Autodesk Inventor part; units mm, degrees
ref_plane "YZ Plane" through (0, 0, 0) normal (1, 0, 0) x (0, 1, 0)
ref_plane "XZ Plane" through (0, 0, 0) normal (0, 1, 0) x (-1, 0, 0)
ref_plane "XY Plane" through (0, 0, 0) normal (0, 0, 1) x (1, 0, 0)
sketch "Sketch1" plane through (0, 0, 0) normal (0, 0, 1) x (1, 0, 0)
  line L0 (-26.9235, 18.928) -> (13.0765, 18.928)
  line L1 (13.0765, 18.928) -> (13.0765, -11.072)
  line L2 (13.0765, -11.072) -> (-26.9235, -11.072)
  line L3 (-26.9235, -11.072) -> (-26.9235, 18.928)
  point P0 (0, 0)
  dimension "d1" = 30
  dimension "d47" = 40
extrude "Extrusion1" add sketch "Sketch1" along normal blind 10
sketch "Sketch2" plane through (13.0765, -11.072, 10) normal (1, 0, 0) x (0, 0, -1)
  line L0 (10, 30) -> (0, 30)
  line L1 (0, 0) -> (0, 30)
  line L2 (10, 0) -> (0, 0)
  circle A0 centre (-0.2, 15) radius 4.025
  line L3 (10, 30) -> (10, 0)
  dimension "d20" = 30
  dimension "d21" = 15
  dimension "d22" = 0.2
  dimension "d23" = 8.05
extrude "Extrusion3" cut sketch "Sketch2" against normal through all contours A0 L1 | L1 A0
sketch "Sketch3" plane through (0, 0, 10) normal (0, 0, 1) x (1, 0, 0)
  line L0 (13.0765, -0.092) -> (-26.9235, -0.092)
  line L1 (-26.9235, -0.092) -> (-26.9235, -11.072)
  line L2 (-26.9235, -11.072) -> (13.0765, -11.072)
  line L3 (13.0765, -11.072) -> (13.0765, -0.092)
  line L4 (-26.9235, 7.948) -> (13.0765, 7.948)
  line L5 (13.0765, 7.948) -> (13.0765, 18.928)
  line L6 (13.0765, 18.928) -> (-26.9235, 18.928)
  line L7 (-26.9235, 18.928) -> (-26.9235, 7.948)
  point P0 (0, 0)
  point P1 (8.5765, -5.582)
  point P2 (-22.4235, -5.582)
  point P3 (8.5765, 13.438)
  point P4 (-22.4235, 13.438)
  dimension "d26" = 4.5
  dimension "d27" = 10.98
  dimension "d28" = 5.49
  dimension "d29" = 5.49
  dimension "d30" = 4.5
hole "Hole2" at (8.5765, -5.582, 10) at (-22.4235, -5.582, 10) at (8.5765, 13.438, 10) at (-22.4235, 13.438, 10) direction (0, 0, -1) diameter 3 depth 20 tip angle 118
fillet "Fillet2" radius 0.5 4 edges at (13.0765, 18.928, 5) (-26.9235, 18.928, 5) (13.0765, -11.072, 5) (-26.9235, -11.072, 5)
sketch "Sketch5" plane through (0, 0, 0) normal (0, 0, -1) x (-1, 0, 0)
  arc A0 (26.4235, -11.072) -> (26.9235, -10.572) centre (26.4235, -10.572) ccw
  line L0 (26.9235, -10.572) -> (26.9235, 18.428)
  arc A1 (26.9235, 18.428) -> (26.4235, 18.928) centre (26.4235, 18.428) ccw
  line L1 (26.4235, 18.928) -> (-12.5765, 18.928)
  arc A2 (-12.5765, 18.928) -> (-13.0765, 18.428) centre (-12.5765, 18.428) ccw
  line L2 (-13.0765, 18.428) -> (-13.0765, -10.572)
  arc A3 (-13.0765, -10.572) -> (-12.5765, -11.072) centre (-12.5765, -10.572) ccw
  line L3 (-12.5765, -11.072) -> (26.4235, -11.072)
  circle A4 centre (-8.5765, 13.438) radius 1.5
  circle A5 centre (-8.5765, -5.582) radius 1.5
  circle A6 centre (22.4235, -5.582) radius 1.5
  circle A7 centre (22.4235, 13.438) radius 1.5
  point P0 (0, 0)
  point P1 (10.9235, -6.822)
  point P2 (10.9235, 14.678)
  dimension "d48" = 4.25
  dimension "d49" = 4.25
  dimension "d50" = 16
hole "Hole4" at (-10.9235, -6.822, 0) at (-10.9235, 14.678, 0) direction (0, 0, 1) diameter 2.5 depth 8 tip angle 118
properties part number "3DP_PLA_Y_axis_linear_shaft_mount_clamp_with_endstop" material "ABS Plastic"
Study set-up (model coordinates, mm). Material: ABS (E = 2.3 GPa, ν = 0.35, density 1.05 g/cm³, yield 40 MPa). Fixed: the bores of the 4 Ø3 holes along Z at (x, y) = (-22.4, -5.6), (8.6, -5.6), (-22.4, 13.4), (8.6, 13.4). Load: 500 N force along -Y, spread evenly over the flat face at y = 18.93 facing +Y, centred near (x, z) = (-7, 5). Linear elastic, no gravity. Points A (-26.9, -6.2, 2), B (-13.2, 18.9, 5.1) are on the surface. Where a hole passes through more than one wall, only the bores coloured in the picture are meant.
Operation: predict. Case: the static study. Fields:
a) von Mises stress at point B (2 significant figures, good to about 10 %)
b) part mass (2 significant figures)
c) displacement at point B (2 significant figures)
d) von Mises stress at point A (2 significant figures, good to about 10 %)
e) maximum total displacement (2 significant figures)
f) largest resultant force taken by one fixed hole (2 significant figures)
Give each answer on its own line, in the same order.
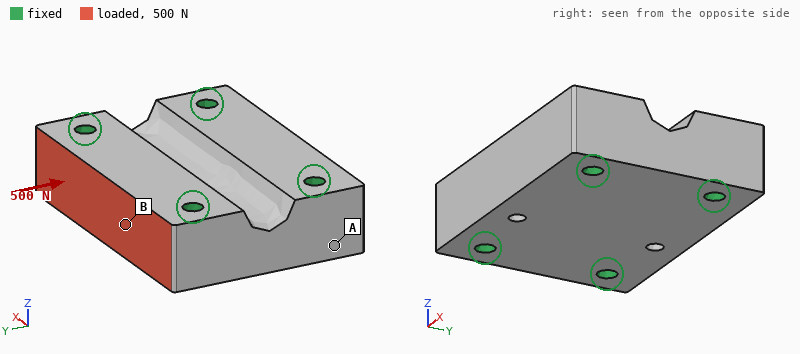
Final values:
1.4 MPa
11 g
14 µm
0.55 MPa
19 µm
190 N
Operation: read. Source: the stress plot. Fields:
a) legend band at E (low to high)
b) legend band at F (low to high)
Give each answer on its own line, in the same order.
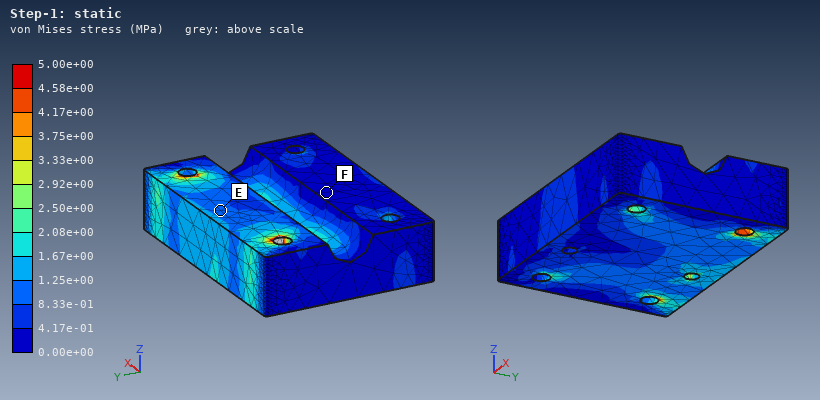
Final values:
8.33e-01 to 1.25e+00 MPa
0.00e+00 to 4.17e-01 MPa
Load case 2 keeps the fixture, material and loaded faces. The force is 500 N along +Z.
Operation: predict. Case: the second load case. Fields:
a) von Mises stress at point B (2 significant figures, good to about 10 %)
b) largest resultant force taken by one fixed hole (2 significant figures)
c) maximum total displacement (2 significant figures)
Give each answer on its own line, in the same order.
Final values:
5.2 MPa
270 N
74 µm
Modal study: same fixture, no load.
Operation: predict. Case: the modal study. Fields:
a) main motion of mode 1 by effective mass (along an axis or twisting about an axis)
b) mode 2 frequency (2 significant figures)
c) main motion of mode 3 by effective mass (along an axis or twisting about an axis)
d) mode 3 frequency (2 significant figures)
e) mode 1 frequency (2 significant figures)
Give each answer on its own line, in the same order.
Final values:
along Z
11 kHz
along Y
12 kHz
9300 Hz
